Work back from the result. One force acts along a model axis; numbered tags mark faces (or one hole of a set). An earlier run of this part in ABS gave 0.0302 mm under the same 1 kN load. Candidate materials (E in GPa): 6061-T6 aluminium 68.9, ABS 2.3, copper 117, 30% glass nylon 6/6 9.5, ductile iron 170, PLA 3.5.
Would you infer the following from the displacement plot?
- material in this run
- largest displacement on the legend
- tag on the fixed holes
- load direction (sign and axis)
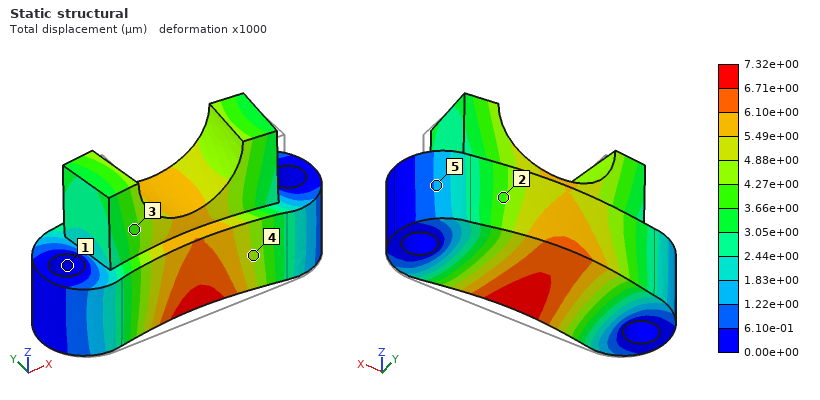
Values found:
30% glass nylon 6/6
7.32e+00 µm
1
+Y
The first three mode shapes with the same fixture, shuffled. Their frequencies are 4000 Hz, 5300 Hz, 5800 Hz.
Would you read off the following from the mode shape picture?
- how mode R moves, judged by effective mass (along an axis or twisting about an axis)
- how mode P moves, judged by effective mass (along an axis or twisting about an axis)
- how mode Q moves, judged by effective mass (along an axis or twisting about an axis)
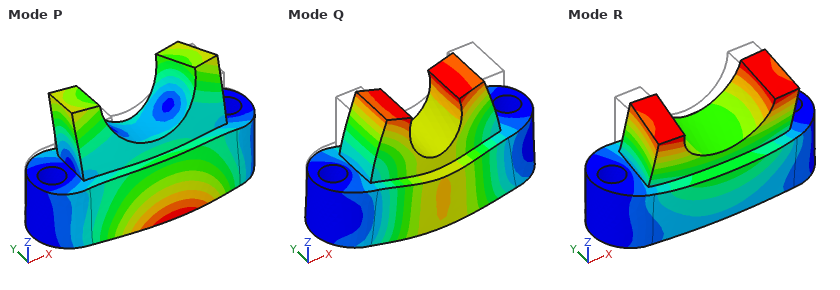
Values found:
along Y
along Y
along Z
